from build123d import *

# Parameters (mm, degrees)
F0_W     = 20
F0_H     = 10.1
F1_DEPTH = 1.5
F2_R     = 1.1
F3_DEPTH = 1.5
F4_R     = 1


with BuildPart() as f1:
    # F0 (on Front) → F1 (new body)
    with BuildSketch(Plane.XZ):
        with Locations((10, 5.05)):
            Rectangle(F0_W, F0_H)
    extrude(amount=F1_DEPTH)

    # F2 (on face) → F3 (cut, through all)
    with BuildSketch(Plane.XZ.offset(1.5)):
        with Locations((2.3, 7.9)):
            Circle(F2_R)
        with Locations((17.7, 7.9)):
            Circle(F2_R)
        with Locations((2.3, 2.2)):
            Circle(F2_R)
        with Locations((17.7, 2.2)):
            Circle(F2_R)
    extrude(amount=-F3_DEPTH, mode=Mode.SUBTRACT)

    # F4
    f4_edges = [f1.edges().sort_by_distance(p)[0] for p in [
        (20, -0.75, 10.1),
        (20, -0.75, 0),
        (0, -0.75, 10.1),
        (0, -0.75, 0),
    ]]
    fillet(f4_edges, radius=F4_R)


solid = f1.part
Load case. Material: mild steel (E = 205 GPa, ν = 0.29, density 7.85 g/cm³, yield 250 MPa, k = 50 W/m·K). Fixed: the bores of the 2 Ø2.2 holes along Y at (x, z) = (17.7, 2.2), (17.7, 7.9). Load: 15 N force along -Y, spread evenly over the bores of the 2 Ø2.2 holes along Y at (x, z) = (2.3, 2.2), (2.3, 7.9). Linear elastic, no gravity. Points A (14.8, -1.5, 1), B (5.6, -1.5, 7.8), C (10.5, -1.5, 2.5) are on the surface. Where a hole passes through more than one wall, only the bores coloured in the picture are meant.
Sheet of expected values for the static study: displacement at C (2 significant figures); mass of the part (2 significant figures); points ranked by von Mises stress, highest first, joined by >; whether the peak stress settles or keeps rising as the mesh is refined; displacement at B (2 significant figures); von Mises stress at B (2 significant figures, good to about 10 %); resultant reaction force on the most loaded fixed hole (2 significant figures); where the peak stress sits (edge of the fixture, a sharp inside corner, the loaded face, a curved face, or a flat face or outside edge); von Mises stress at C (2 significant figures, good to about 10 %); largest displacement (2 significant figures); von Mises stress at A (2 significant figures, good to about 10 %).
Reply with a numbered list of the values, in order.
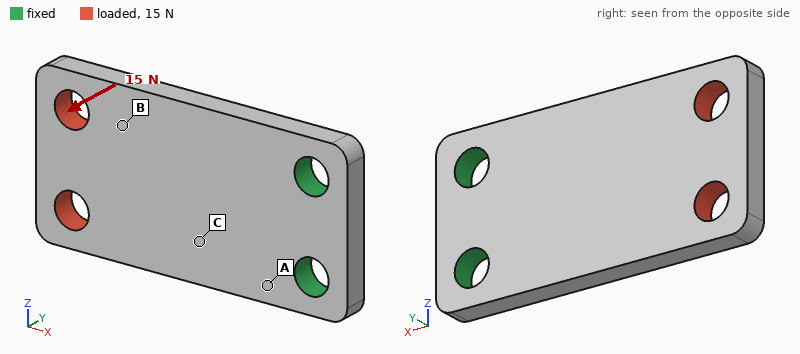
1. 7.0 µm
2. 2.2 g
3. A > C > B
4. keeps rising
5. 18 µm
6. 13 MPa
7. 7.5 N
8. edge of the fixture
9. 31 MPa
10. 33 µm
11. 48 MPa
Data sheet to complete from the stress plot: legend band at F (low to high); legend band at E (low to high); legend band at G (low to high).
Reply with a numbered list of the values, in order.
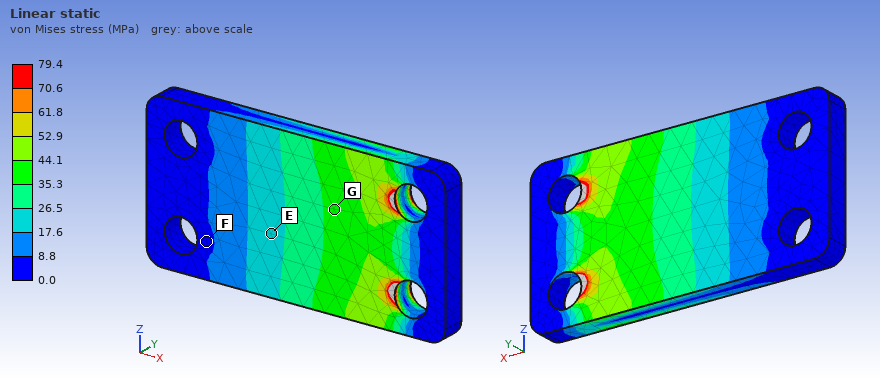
1. 0.0 to 8.8 MPa
2. 17.6 to 26.5 MPa
3. 35.3 to 44.1 MPa
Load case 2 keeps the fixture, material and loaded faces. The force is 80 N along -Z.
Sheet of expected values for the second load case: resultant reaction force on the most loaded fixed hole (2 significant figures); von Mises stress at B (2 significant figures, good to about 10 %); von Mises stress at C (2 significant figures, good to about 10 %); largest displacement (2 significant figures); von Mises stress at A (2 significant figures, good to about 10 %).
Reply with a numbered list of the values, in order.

1. 180 N
2. 12 MPa
3. 17 MPa
4. 5.8 µm
5. 31 MPa
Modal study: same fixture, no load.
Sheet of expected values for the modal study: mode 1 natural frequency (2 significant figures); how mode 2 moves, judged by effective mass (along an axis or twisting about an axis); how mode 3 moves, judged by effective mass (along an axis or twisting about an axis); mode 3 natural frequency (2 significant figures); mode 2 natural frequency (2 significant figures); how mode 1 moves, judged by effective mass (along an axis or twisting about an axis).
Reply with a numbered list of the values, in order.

1. 4600 Hz
2. twisting about X
3. along Z
4. 24 kHz
5. 16 kHz
6. along Y
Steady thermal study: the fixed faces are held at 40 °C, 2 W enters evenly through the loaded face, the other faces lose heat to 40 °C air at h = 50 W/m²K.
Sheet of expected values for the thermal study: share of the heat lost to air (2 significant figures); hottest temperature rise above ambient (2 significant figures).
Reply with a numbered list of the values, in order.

1. 19 %
2. 37 K
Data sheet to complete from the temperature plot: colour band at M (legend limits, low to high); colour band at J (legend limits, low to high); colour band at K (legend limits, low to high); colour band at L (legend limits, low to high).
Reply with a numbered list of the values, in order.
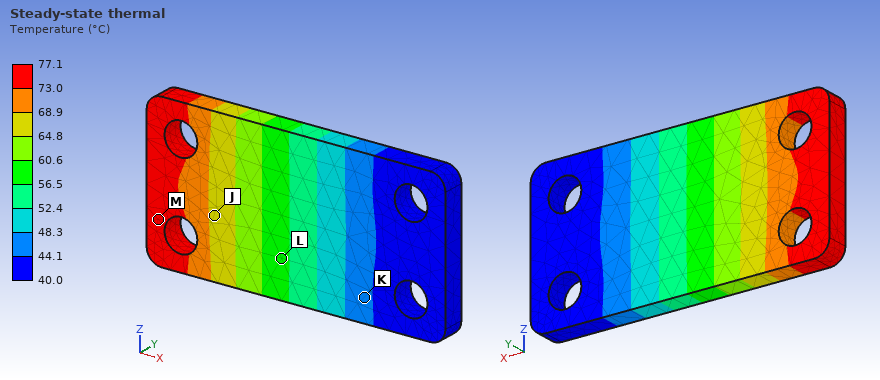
1. 73.0 to 77.1 °C
2. 64.8 to 68.9 °C
3. 44.1 to 48.3 °C
4. 56.5 to 60.6 °C
